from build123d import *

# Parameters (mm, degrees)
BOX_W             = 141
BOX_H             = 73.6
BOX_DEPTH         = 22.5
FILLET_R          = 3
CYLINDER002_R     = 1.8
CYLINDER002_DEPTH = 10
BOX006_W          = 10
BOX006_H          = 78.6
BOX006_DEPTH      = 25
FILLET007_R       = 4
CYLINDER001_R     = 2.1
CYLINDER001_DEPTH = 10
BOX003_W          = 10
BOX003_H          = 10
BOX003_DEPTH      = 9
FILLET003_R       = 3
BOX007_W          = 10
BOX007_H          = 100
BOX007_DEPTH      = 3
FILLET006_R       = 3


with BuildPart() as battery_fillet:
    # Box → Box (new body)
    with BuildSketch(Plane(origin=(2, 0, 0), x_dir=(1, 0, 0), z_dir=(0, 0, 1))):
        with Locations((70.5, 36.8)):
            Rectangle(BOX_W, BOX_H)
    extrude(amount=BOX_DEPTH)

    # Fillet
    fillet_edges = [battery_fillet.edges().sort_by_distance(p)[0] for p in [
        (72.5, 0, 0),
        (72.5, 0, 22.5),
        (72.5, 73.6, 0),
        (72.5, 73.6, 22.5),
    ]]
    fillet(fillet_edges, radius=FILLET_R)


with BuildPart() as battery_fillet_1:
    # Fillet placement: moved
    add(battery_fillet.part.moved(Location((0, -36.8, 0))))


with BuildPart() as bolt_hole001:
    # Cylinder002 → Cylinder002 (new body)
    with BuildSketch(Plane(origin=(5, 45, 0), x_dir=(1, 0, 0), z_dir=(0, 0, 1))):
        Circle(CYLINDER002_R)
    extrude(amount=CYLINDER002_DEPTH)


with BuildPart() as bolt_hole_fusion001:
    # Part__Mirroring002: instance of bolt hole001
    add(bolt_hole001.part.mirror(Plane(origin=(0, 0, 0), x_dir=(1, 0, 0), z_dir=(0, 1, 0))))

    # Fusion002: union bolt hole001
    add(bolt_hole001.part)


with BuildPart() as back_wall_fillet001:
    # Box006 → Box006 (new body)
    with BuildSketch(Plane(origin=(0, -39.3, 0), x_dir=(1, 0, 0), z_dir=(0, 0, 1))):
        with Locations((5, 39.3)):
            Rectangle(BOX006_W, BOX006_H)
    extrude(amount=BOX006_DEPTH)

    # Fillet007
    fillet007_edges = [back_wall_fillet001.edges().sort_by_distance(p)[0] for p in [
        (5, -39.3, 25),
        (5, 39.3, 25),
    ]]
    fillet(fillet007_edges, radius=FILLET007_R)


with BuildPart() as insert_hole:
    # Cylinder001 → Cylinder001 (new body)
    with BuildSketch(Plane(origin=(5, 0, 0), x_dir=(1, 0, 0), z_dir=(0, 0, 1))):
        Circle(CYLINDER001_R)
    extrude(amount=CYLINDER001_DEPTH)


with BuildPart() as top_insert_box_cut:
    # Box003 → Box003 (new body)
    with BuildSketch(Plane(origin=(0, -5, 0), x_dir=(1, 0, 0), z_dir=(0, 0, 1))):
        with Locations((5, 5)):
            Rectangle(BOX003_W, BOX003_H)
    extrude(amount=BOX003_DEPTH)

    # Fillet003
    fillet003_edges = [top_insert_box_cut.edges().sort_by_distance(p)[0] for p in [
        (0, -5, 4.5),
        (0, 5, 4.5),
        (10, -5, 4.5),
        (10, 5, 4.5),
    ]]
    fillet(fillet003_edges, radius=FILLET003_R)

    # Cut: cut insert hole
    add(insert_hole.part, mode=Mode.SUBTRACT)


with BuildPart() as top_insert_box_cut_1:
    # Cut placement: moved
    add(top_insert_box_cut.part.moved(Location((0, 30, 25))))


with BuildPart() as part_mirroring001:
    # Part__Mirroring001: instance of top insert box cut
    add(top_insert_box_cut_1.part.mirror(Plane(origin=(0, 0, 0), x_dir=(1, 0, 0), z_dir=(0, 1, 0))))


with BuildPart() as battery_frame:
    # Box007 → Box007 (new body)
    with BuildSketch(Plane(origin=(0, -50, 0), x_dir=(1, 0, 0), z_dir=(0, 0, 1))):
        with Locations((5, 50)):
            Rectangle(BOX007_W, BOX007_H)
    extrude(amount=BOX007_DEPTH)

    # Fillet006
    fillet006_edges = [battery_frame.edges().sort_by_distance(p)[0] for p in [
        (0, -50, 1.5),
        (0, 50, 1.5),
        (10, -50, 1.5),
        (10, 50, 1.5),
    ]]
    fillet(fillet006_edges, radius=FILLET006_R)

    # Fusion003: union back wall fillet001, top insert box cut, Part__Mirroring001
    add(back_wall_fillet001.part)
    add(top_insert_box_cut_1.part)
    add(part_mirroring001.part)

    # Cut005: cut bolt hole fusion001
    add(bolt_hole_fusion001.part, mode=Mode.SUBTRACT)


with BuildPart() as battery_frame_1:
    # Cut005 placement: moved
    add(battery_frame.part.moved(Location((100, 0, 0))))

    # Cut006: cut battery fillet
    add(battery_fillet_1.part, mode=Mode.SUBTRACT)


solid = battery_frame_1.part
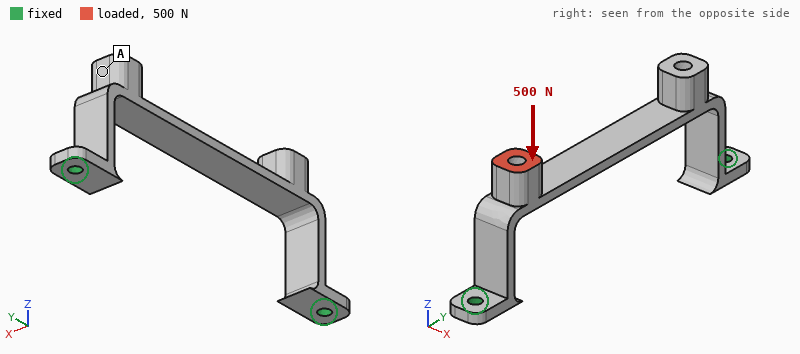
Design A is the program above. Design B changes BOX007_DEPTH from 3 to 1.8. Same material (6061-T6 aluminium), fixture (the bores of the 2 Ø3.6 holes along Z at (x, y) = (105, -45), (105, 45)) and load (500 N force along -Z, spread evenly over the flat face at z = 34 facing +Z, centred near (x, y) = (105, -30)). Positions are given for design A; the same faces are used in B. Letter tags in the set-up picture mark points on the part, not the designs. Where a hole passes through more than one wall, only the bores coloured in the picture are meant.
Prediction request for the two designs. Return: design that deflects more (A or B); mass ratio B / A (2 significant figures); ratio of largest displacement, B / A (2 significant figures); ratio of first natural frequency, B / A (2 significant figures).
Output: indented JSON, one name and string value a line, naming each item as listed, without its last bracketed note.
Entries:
{
  "design that deflects more": "B",
  "mass ratio B / A": "0.96",
  "ratio of largest displacement, B / A": "1.3",
  "ratio of first natural frequency, B / A": "0.68"
}
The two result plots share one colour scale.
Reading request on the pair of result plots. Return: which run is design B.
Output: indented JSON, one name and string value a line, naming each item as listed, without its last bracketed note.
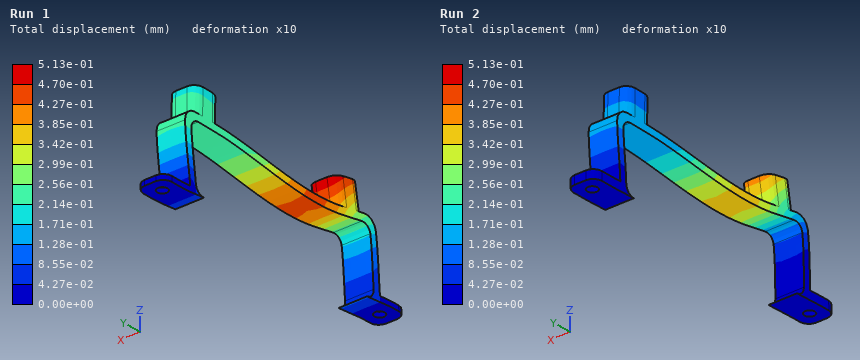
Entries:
{
  "which run is design B": "Run 1"
}
